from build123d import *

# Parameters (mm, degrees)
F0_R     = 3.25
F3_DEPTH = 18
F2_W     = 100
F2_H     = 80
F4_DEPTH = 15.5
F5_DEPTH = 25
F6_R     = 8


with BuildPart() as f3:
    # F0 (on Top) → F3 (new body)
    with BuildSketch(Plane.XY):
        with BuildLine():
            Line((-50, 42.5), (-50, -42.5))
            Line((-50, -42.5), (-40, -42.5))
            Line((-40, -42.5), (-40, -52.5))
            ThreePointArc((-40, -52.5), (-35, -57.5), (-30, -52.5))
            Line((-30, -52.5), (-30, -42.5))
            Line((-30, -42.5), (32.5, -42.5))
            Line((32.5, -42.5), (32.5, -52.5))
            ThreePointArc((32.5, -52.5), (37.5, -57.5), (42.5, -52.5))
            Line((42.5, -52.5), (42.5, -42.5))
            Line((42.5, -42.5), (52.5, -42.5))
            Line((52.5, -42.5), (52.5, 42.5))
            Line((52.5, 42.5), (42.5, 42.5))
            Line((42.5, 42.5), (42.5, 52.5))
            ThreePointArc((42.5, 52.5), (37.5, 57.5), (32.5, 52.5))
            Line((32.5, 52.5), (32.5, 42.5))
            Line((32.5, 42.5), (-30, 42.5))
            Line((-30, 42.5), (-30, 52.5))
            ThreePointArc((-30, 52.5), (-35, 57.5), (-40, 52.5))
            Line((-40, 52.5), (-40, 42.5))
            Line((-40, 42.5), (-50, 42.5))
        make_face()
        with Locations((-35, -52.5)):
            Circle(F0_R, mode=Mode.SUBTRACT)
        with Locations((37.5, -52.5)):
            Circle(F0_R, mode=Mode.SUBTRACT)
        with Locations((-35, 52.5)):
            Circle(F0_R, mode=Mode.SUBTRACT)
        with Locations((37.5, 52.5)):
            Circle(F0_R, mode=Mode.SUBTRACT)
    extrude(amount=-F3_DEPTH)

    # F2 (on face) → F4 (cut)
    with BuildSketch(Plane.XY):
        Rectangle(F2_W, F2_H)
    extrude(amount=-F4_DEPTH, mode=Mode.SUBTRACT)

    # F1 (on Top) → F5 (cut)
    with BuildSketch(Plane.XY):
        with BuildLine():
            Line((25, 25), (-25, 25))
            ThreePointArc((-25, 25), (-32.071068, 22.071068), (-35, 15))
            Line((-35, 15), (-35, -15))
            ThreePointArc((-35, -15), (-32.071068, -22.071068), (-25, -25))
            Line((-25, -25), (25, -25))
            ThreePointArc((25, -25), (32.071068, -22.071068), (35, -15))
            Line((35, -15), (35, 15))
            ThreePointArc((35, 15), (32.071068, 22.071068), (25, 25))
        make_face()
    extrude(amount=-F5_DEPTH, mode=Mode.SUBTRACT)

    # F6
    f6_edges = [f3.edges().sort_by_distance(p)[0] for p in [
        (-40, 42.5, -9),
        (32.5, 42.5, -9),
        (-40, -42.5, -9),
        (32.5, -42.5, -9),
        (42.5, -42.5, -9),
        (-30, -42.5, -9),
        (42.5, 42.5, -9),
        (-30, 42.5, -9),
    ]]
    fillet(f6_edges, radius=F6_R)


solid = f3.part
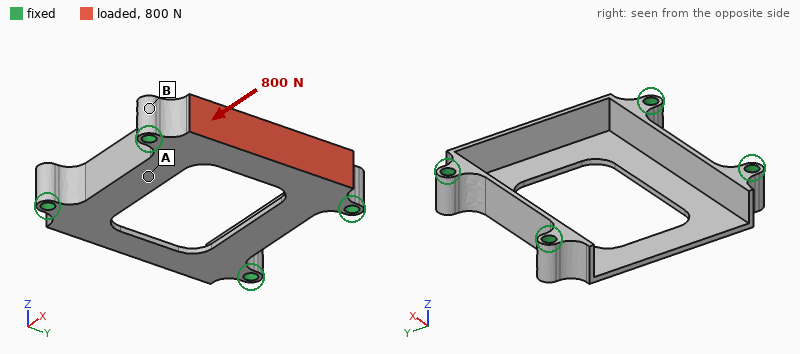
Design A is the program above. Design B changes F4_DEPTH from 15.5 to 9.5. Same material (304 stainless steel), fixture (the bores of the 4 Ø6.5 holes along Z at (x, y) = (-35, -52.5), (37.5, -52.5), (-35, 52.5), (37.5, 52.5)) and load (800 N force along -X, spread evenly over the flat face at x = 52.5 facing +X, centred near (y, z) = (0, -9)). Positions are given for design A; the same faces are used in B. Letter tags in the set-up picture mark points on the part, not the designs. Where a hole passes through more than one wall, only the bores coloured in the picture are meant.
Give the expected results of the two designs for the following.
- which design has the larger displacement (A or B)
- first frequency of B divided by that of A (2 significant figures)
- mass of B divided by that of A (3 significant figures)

A
2.4
1.81
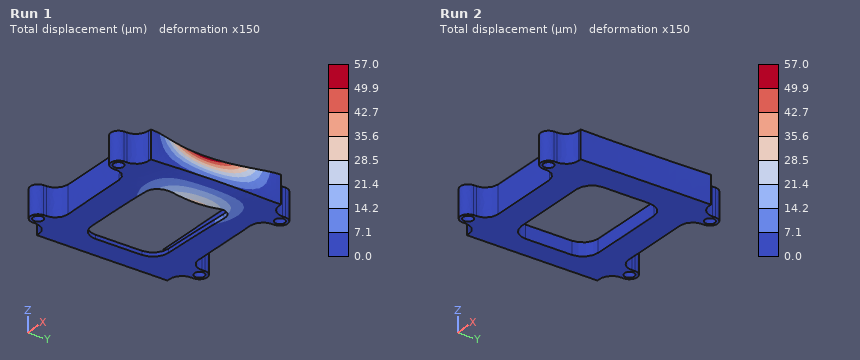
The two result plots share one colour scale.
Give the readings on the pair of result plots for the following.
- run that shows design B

Run 2
